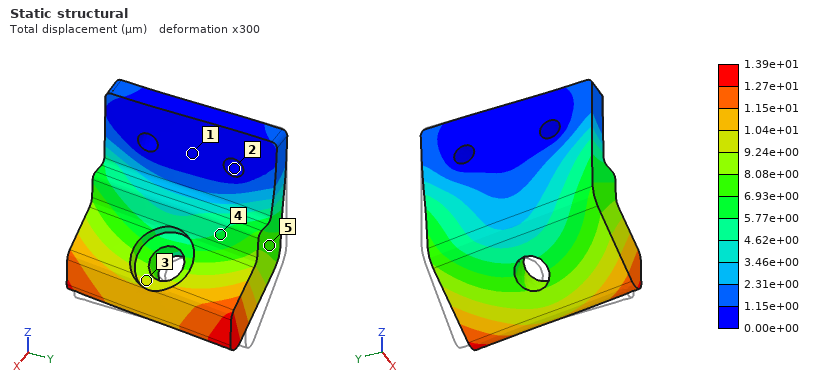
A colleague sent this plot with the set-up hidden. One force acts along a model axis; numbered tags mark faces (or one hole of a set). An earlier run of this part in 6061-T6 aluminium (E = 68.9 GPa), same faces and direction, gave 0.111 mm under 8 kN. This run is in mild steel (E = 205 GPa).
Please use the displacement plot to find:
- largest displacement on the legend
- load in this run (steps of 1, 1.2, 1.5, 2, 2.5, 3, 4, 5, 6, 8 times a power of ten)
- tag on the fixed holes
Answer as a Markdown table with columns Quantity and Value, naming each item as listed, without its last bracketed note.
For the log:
| Quantity | Value |
|---|---|
| largest displacement on the legend | 1.39e+01 µm |
| load in this run | 3 kN |
| tag on the fixed holes | 2 |
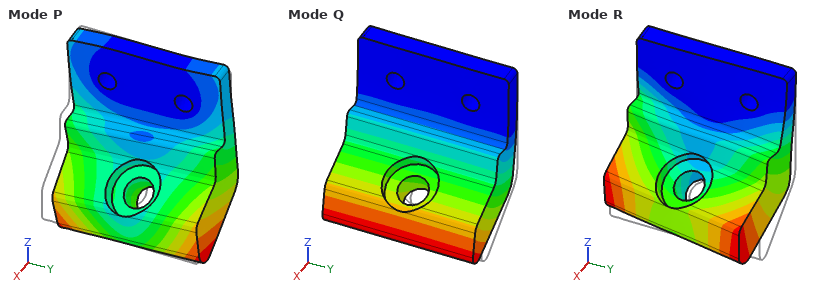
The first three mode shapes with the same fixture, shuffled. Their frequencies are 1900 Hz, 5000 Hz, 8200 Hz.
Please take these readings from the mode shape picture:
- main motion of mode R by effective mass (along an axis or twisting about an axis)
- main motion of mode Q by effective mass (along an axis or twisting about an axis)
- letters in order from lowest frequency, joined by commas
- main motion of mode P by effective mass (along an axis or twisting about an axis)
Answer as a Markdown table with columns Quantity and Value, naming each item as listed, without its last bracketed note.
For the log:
| Quantity | Value |
|---|---|
| main motion of mode R by effective mass | along Y |
| main motion of mode Q by effective mass | along X |
| letters in order from lowest frequency, joined by commas | Q, R, P |
| main motion of mode P by effective mass | along Y |
